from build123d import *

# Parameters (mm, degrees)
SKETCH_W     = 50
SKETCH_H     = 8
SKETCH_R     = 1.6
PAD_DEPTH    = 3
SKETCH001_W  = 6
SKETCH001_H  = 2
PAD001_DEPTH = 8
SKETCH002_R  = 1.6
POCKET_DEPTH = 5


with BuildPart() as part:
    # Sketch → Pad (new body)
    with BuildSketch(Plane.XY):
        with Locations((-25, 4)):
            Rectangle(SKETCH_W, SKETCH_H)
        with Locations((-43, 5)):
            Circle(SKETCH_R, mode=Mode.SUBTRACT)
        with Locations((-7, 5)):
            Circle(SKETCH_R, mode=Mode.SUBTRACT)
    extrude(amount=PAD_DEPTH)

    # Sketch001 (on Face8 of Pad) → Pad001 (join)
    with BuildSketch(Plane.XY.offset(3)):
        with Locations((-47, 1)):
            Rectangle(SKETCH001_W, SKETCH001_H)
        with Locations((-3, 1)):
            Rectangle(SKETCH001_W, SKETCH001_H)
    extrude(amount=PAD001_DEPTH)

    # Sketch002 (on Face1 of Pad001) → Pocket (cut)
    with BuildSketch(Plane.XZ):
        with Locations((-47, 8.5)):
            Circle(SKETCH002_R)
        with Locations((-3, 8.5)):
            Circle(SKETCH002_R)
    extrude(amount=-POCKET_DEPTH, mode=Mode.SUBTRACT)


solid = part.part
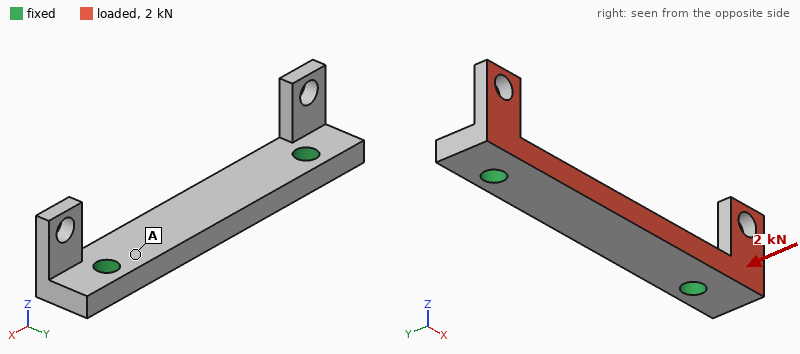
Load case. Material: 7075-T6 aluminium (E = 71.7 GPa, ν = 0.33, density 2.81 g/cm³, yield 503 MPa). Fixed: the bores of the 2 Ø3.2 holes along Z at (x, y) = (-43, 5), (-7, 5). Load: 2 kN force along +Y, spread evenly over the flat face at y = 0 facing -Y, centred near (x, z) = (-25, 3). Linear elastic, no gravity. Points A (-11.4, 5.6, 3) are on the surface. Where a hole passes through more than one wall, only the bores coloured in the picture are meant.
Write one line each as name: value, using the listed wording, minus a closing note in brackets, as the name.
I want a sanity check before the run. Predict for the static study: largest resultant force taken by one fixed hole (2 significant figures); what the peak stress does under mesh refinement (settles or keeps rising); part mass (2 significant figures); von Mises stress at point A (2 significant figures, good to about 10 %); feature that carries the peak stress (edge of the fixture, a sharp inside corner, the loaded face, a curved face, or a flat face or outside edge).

largest resultant force taken by one fixed hole: 1.0 kN
what the peak stress does under mesh refinement: keeps rising
part mass: 3.7 g
von Mises stress at point A: 35 MPa
feature that carries the peak stress: a sharp inside corner
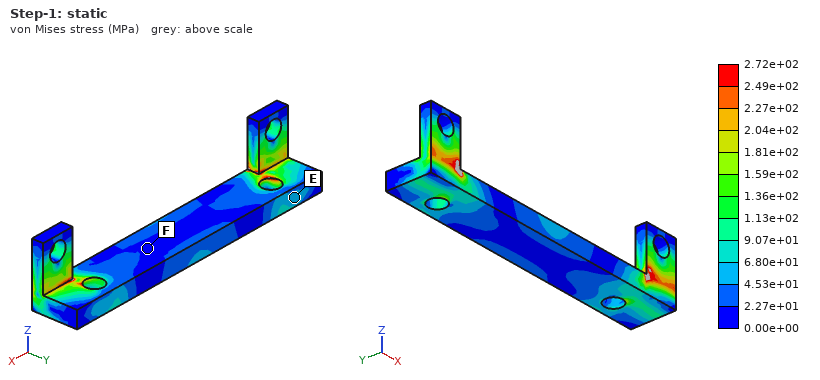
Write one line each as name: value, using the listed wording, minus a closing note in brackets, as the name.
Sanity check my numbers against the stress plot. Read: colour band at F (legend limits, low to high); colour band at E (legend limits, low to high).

colour band at F: 0.00e+00 to 2.27e+01 MPa
colour band at E: 4.53e+01 to 6.80e+01 MPa
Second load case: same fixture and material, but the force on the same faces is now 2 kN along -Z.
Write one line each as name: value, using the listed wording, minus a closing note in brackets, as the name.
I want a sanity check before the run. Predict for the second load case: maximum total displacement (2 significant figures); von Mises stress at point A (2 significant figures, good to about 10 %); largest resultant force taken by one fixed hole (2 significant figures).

maximum total displacement: 0.13 mm
von Mises stress at point A: 140 MPa
largest resultant force taken by one fixed hole: 1.0 kN
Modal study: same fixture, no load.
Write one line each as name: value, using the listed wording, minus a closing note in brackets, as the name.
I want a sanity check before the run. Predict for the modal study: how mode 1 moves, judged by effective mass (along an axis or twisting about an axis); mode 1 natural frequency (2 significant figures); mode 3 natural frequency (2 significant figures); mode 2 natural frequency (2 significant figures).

how mode 1 moves, judged by effective mass: along Z
mode 1 natural frequency: 13 kHz
mode 3 natural frequency: 19 kHz
mode 2 natural frequency: 19 kHz
